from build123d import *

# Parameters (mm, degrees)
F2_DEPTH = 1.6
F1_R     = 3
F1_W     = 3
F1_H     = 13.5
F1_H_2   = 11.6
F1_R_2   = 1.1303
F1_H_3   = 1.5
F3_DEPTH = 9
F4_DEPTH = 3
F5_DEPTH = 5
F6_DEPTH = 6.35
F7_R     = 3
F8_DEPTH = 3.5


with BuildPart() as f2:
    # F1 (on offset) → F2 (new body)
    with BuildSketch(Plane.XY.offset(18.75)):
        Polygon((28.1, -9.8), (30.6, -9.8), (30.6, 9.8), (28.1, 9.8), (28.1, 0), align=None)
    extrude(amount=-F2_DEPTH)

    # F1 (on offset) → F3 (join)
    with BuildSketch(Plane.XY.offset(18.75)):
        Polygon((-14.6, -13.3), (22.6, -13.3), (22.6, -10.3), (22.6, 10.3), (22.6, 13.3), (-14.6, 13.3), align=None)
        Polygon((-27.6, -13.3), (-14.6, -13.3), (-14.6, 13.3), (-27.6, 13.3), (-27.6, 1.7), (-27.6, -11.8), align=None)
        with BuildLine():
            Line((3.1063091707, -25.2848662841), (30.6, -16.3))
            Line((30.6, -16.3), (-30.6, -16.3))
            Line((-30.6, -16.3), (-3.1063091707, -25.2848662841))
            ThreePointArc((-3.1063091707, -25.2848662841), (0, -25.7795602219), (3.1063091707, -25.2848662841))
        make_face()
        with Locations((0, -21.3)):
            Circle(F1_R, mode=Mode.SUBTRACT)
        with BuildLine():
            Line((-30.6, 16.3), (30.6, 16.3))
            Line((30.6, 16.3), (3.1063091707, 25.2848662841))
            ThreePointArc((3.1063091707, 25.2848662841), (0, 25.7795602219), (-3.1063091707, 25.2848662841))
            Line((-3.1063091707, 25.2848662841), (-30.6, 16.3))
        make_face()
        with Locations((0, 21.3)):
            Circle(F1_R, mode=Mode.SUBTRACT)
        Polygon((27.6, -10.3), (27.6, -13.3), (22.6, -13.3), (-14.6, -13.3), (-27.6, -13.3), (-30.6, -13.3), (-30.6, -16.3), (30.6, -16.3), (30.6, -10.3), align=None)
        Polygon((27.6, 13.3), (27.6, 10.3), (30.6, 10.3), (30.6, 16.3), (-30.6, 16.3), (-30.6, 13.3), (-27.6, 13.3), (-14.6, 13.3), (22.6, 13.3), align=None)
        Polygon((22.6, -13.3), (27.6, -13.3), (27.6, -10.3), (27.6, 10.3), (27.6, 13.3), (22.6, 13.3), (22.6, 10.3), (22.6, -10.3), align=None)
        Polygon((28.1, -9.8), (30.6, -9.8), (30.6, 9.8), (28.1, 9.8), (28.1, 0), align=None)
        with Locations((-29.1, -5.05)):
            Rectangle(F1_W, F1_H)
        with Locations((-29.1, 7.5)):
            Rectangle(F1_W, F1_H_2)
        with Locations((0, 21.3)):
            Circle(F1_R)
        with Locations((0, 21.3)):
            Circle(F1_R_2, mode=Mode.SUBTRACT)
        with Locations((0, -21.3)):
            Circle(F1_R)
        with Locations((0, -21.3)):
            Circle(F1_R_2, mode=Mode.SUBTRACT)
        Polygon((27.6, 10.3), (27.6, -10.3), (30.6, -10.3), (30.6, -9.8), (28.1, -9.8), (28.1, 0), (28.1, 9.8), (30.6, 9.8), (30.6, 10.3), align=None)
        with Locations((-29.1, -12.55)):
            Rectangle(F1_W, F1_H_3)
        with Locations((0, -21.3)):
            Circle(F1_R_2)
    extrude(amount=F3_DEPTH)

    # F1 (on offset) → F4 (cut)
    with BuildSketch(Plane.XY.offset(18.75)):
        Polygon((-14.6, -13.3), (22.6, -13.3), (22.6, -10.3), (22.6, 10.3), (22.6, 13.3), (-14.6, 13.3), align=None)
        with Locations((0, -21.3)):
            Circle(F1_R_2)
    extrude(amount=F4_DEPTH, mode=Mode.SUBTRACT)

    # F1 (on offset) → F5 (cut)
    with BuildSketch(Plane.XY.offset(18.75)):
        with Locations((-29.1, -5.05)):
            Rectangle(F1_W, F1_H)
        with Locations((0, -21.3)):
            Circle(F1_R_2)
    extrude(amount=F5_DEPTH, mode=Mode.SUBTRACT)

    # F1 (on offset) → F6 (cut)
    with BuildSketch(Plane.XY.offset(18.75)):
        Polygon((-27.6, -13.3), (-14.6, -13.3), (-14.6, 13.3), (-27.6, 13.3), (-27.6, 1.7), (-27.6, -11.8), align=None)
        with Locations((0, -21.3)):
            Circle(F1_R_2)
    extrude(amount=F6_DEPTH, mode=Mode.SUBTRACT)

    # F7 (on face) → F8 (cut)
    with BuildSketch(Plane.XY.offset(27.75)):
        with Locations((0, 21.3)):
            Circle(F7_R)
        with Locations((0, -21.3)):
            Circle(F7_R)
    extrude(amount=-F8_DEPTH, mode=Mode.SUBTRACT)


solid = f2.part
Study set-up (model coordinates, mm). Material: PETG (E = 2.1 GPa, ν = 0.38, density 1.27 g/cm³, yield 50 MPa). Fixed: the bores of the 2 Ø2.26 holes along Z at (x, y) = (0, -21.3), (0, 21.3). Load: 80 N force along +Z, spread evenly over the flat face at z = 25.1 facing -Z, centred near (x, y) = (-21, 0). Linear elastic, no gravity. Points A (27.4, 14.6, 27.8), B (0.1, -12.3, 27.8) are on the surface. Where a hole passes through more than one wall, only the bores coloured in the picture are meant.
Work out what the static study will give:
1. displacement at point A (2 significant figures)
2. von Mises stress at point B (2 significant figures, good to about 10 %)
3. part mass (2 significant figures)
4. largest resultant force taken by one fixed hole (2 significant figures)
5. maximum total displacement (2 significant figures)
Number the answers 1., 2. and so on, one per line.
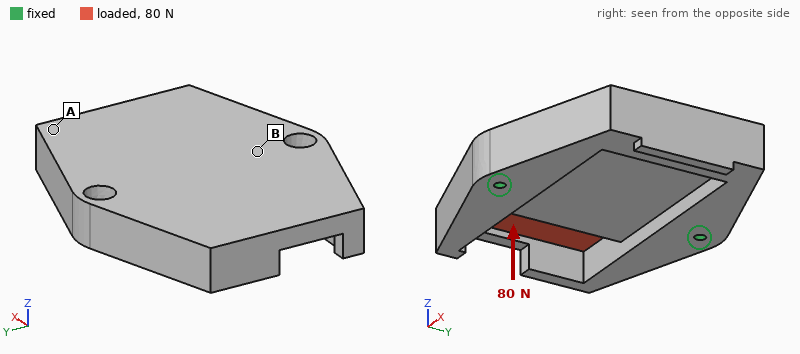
1. 0.19 mm
2. 2.5 MPa
3. 23 g
4. 66 N
5. 0.44 mm
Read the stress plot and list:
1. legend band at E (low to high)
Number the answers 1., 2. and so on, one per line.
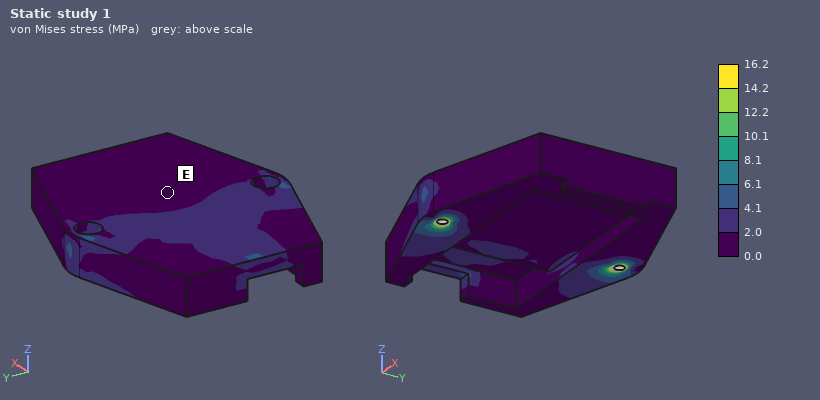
1. 0.0 to 2.0 MPa
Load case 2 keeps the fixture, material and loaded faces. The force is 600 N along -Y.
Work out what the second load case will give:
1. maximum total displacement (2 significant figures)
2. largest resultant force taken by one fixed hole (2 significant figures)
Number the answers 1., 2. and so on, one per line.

1. 0.29 mm
2. 420 N
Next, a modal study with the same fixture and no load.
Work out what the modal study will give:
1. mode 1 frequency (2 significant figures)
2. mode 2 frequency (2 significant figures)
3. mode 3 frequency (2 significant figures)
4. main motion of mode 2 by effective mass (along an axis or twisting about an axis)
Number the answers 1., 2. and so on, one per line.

1. 850 Hz
2. 1700 Hz
3. 2200 Hz
4. along Z
